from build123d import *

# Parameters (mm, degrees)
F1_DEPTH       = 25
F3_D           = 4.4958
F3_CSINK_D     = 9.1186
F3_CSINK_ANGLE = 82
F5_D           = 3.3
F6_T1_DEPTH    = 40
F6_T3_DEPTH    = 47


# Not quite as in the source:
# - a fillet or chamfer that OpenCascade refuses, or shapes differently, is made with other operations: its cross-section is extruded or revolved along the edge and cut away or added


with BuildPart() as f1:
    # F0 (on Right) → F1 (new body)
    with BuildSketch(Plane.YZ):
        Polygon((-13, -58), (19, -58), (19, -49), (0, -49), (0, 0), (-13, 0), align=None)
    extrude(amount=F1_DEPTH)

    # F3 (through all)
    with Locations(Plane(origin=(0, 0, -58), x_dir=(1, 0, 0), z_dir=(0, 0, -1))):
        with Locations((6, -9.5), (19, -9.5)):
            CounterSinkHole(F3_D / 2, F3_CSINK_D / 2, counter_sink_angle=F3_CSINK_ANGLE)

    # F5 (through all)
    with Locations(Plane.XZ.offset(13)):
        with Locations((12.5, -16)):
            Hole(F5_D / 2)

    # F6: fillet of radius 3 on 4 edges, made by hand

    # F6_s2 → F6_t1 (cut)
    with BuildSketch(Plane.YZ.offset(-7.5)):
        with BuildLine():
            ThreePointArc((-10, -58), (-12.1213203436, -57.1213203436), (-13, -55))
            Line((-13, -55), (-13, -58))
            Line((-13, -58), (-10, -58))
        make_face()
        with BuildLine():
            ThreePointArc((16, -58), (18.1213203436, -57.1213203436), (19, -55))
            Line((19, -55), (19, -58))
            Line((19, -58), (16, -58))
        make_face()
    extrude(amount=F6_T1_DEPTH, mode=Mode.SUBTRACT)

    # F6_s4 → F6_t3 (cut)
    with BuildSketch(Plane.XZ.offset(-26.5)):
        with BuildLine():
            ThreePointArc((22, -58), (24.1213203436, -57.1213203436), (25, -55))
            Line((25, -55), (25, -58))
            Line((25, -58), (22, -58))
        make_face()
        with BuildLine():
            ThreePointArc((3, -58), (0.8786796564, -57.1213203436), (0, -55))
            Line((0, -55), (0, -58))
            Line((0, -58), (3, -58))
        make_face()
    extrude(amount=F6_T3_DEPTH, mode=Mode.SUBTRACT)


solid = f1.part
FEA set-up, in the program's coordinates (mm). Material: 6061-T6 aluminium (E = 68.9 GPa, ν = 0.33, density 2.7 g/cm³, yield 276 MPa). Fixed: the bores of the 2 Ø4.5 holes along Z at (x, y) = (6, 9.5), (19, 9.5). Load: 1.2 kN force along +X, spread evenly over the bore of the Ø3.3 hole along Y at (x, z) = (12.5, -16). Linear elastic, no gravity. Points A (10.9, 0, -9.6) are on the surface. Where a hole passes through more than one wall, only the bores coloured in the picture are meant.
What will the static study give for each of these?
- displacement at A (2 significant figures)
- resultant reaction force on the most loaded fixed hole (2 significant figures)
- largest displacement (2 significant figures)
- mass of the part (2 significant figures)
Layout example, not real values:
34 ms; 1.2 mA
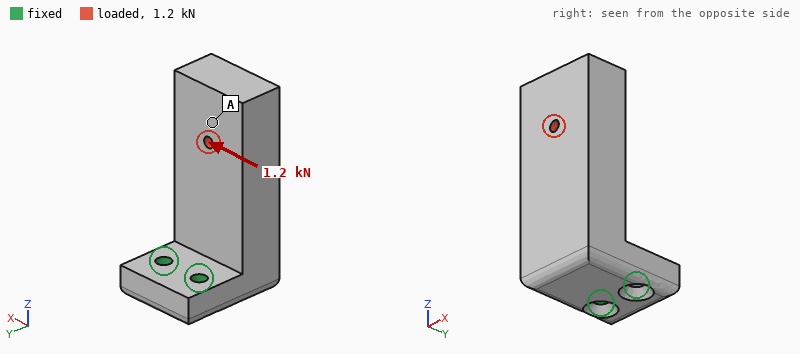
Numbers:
0.16 mm; 2.7 kN; 0.19 mm; 60 g
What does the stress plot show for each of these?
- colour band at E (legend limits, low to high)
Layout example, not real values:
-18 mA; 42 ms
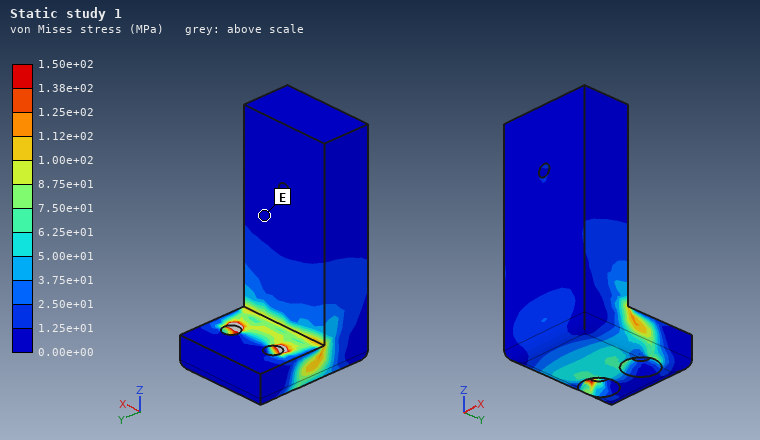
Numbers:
0.00e+00 to 1.25e+01 MPa
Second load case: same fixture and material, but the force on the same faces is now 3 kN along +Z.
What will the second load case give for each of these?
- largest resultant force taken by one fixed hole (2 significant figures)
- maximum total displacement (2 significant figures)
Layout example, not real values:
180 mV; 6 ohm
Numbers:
1.5 kN; 0.28 mm
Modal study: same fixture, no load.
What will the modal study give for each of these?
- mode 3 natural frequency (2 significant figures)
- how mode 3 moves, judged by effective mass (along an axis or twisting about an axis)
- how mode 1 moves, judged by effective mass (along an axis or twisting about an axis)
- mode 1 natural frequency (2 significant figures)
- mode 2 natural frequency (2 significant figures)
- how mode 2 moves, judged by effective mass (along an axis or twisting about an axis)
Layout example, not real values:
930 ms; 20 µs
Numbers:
8100 Hz; along Z; along Y; 1700 Hz; 2600 Hz; along X
